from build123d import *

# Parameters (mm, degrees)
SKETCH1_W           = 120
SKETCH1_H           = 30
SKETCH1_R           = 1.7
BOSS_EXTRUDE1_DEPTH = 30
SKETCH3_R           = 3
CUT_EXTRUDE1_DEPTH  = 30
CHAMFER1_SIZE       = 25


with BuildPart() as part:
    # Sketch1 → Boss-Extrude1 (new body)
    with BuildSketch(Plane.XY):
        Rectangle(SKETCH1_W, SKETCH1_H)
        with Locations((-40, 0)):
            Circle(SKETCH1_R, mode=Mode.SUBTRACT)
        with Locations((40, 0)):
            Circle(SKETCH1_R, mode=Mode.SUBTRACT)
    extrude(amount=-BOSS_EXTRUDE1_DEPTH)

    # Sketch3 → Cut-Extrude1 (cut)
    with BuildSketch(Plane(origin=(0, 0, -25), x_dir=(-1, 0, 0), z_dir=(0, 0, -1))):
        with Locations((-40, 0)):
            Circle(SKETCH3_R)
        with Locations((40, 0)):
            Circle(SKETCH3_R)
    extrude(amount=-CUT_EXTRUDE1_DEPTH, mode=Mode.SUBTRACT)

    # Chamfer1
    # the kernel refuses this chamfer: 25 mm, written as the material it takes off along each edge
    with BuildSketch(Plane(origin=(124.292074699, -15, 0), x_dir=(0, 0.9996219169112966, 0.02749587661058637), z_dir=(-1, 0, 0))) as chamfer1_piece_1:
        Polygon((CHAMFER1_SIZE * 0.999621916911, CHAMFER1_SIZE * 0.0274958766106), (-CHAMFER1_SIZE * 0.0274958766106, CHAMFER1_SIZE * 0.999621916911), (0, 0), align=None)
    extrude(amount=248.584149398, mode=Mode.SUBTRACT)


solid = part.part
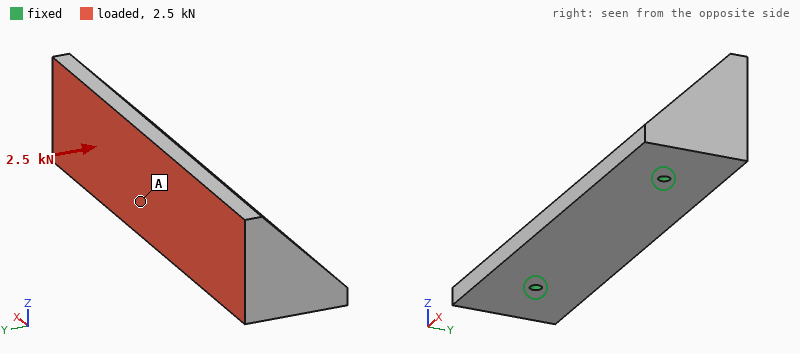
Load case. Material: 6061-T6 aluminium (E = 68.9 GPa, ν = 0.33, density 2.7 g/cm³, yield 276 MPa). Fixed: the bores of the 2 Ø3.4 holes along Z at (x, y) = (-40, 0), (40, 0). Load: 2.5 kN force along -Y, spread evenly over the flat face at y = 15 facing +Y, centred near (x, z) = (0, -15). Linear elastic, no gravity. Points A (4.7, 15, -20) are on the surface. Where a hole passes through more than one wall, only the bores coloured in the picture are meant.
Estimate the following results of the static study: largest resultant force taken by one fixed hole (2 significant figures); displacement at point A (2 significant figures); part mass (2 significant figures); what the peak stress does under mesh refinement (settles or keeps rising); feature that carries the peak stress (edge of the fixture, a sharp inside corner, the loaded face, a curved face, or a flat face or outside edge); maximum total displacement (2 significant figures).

1.3 kN
0.054 mm
190 g
keeps rising
edge of the fixture
0.10 mm
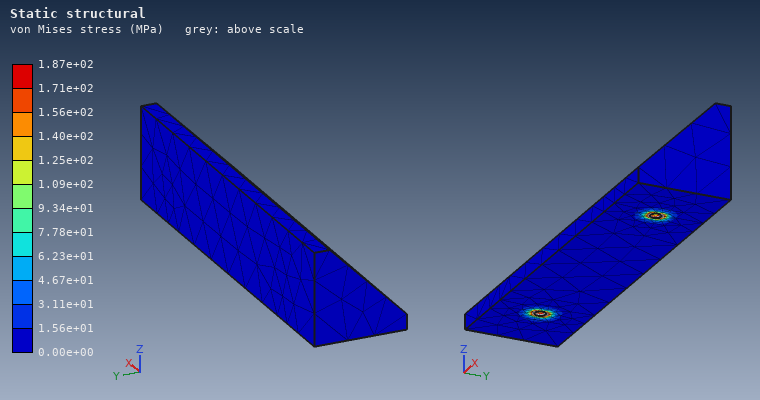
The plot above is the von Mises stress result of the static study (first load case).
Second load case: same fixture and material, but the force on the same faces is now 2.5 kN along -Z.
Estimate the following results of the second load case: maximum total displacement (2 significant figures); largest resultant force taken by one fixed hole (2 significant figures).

0.12 mm
1.3 kN
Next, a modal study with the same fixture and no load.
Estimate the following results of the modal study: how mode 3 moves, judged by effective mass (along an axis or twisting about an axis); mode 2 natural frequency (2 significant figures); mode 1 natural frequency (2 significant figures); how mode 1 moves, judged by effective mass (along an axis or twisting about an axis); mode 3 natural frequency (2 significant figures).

twisting about Z
6700 Hz
2500 Hz
along Y
7100 Hz
